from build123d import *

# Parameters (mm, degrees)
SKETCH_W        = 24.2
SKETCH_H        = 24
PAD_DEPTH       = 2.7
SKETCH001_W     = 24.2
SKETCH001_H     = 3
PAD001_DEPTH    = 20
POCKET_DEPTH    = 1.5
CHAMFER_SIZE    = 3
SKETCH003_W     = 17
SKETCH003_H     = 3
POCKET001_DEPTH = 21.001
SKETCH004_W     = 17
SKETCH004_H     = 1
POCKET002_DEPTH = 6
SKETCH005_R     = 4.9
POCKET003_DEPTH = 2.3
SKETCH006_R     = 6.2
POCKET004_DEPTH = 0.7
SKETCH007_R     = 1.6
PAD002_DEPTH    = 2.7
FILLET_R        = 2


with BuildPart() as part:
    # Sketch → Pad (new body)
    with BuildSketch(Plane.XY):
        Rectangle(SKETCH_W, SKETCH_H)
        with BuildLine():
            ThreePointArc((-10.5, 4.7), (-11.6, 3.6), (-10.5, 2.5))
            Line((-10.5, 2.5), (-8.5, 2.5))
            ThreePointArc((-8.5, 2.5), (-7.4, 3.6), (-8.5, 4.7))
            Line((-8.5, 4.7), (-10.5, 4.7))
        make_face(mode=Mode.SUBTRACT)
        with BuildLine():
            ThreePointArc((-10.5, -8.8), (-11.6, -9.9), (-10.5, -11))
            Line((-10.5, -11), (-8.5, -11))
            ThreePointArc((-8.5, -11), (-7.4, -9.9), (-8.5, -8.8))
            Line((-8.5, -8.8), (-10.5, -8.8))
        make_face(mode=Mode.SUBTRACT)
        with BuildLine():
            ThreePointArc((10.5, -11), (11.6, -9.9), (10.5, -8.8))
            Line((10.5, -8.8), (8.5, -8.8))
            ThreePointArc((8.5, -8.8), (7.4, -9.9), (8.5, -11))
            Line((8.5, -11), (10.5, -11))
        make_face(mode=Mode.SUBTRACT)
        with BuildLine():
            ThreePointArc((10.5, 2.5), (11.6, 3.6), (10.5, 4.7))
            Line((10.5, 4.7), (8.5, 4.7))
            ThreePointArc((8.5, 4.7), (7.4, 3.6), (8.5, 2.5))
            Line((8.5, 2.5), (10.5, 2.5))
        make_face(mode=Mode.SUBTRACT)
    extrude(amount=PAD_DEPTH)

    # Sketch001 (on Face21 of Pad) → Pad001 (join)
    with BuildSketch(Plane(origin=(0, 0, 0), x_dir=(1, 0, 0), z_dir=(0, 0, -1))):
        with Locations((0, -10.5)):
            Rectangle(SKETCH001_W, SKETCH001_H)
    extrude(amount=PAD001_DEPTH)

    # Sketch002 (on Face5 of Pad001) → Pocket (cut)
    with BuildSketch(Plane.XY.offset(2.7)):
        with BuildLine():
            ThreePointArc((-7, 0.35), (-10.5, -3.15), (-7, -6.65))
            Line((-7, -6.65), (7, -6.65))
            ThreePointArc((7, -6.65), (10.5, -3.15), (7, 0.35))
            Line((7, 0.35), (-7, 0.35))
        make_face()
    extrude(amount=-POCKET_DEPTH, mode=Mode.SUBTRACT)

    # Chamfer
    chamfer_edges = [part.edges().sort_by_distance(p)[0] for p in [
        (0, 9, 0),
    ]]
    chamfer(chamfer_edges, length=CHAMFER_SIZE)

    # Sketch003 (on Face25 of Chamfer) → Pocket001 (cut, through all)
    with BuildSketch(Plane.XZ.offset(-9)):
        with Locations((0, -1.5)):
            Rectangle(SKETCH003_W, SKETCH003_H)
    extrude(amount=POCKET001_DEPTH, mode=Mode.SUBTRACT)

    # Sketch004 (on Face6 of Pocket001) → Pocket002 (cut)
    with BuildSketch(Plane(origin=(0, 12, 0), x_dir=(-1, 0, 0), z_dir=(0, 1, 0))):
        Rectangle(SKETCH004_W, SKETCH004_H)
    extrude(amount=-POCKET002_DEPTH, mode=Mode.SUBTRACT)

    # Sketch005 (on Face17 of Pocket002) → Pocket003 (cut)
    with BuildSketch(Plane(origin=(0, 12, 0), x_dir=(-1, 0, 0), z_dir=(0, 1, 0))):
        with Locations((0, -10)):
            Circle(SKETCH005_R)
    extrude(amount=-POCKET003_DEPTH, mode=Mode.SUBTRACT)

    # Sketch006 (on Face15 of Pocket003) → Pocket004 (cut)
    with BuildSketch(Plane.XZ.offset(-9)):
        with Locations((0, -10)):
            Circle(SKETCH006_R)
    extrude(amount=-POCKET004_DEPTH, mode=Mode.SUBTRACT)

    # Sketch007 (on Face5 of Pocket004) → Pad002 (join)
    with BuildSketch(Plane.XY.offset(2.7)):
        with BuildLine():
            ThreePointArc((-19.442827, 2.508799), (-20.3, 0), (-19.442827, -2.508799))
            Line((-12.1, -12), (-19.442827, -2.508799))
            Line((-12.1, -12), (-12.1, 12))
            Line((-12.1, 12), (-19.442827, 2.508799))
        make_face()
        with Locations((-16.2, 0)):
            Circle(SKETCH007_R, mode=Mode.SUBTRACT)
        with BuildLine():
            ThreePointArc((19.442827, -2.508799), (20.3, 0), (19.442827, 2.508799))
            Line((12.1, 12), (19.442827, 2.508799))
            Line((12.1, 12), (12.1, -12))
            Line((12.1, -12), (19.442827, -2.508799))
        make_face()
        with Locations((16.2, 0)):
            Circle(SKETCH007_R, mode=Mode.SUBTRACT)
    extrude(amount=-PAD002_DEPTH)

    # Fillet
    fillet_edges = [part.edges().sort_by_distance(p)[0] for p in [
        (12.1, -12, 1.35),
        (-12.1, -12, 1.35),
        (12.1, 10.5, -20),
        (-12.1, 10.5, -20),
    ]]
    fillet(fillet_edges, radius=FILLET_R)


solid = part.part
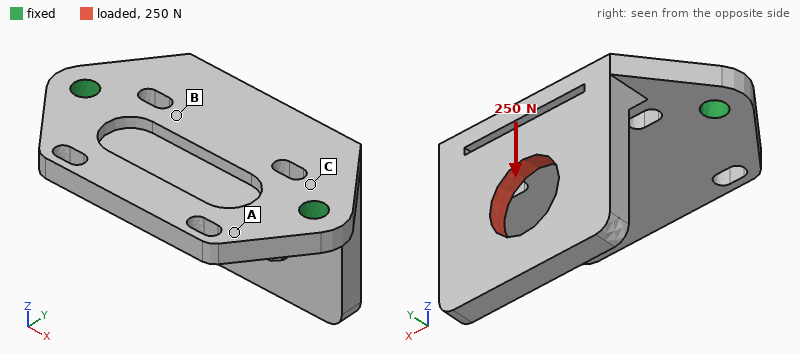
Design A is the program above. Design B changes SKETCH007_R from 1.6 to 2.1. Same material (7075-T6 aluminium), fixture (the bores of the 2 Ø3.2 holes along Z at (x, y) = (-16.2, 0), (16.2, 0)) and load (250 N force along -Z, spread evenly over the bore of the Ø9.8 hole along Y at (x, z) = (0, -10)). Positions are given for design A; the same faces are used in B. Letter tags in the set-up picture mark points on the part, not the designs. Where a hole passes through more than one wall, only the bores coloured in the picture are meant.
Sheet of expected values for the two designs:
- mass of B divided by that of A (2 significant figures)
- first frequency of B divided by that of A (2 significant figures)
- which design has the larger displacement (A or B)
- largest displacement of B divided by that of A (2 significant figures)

0.99
1.0
A
0.90
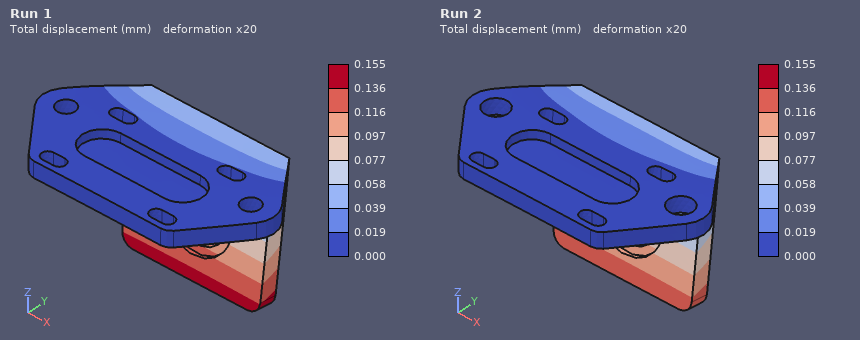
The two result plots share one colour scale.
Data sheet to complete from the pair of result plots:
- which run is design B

Run 2
